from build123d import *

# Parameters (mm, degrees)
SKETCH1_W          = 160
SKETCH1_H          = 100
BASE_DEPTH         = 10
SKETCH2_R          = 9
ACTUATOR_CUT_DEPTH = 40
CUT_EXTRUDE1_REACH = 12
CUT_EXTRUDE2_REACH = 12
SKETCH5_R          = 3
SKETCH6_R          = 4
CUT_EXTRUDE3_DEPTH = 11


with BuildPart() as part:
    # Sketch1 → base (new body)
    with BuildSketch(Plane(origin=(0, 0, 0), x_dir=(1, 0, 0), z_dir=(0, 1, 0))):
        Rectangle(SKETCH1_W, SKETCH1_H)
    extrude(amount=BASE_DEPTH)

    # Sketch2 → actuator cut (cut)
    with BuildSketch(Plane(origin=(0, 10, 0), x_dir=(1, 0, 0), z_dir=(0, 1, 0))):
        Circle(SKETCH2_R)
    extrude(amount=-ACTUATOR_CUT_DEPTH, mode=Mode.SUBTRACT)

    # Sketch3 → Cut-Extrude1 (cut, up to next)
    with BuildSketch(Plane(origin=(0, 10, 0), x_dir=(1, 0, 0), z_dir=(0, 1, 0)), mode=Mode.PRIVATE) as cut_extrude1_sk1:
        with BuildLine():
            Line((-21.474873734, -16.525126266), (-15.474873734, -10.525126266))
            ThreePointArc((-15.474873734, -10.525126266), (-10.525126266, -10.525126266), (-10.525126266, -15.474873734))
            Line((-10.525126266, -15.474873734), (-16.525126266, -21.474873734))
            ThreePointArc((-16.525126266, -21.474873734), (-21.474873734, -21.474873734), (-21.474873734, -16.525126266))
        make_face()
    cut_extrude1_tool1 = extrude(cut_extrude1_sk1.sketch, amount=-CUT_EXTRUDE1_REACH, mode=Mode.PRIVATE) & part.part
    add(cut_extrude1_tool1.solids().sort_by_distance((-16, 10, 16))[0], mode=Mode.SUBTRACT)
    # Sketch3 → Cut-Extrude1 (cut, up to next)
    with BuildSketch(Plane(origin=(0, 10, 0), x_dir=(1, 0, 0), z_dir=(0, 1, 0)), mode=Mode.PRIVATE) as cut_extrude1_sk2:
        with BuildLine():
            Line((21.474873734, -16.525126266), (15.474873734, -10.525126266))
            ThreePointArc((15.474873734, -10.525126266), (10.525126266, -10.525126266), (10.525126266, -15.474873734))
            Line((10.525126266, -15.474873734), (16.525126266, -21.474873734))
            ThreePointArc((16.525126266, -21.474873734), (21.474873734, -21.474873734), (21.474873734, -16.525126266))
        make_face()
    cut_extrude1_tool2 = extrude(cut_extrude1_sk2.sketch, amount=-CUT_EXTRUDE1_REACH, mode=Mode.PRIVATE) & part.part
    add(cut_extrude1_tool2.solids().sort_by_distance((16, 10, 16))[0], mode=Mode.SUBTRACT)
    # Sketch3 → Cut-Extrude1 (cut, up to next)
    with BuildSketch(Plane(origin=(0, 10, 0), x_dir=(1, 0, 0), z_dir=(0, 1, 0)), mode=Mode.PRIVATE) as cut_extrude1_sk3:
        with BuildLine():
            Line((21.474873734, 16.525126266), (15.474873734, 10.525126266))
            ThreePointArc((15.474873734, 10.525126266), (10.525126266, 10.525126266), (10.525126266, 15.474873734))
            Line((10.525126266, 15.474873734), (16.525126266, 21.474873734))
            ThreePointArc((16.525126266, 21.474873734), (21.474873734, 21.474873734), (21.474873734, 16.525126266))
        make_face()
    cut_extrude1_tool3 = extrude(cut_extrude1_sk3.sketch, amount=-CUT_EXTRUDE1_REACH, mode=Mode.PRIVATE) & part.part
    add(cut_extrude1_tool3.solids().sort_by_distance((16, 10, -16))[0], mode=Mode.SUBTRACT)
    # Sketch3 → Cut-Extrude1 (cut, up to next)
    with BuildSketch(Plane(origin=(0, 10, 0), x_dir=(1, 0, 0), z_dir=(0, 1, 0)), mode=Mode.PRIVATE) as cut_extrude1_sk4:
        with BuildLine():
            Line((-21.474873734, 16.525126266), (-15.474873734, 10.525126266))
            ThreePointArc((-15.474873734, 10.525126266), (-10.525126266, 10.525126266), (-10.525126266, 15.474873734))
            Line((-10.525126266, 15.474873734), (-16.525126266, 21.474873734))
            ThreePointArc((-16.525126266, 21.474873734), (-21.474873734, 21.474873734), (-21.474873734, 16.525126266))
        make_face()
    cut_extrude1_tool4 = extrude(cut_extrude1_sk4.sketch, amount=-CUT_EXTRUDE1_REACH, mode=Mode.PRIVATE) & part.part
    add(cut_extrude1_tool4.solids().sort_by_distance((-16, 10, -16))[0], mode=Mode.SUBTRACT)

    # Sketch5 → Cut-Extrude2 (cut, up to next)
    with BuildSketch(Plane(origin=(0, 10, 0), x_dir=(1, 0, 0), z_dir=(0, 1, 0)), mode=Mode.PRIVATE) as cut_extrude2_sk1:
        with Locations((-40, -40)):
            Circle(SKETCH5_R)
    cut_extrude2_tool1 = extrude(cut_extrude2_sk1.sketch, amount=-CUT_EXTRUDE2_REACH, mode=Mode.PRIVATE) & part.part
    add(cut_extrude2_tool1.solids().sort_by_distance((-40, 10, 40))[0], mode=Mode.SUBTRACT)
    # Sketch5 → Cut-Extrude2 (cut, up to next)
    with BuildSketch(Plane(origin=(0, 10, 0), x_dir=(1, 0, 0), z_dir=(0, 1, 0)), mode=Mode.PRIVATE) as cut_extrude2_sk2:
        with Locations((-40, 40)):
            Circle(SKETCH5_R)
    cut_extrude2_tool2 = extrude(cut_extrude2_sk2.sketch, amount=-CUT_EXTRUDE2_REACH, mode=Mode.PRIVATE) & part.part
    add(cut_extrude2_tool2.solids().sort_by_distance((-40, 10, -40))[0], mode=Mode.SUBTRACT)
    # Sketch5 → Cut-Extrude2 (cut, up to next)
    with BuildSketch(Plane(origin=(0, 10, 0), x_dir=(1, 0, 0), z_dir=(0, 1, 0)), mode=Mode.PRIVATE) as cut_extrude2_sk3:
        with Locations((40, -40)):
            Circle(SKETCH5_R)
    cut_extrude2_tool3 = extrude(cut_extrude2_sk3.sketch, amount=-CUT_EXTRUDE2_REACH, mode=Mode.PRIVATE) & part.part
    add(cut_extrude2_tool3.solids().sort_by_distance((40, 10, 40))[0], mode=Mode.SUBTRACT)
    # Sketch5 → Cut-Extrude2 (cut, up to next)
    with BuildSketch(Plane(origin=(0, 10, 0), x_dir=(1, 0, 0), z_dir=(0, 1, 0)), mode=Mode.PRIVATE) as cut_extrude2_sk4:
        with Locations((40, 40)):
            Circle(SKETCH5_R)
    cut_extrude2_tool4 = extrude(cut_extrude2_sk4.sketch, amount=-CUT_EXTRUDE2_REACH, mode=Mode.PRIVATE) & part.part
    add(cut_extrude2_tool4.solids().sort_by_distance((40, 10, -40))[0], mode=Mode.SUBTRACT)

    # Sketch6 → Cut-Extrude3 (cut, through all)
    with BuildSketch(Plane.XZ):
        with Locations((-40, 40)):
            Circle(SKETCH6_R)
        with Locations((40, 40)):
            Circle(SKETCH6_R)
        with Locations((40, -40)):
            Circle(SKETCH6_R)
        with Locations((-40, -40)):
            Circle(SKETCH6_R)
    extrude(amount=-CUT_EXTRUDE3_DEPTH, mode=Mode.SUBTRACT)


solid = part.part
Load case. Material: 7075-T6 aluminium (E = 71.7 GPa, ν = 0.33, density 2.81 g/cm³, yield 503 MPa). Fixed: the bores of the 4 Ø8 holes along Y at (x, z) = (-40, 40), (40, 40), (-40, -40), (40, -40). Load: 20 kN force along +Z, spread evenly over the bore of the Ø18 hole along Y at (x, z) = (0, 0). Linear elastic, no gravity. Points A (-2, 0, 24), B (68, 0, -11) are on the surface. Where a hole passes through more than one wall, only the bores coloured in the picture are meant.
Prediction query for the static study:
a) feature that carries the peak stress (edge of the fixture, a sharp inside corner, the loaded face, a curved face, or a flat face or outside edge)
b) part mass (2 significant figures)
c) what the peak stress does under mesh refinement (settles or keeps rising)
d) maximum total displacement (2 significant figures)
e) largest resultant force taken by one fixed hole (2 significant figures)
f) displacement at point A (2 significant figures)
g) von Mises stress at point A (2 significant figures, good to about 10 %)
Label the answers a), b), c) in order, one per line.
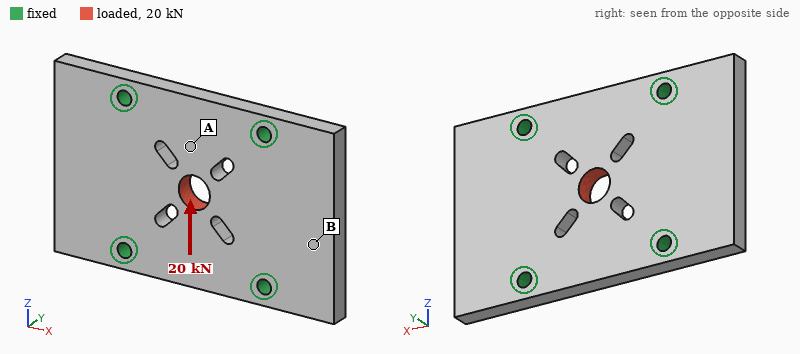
a) edge of the fixture
b) 430 g
c) keeps rising
d) 25 µm
e) 5.7 kN
f) 19 µm
g) 14 MPa
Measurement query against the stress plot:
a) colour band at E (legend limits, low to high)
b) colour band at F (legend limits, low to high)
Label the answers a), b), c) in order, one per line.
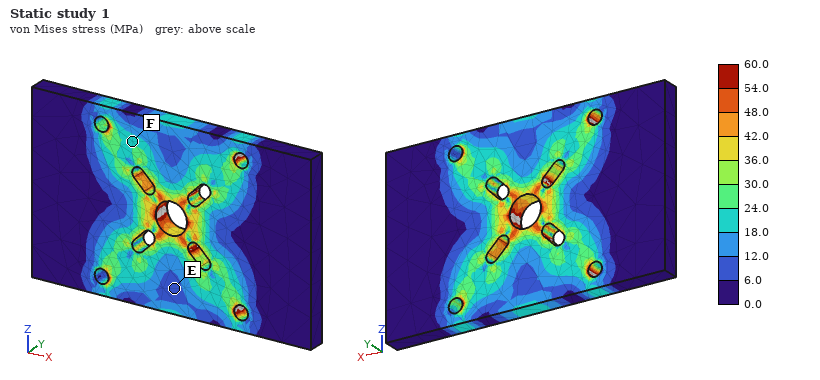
a) 6.0 to 12.0 MPa
b) 18.0 to 24.0 MPa
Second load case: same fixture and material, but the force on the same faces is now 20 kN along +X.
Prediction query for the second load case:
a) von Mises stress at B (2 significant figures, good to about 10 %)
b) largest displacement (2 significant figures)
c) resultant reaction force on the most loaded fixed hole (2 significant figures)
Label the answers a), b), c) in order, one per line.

a) 7.0 MPa
b) 21 µm
c) 5.1 kN
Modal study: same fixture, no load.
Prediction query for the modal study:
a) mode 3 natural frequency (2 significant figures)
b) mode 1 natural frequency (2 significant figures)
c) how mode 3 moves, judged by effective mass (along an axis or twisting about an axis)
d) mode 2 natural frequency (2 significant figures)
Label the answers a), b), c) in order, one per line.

a) 5400 Hz
b) 3800 Hz
c) along Y
d) 3900 Hz
